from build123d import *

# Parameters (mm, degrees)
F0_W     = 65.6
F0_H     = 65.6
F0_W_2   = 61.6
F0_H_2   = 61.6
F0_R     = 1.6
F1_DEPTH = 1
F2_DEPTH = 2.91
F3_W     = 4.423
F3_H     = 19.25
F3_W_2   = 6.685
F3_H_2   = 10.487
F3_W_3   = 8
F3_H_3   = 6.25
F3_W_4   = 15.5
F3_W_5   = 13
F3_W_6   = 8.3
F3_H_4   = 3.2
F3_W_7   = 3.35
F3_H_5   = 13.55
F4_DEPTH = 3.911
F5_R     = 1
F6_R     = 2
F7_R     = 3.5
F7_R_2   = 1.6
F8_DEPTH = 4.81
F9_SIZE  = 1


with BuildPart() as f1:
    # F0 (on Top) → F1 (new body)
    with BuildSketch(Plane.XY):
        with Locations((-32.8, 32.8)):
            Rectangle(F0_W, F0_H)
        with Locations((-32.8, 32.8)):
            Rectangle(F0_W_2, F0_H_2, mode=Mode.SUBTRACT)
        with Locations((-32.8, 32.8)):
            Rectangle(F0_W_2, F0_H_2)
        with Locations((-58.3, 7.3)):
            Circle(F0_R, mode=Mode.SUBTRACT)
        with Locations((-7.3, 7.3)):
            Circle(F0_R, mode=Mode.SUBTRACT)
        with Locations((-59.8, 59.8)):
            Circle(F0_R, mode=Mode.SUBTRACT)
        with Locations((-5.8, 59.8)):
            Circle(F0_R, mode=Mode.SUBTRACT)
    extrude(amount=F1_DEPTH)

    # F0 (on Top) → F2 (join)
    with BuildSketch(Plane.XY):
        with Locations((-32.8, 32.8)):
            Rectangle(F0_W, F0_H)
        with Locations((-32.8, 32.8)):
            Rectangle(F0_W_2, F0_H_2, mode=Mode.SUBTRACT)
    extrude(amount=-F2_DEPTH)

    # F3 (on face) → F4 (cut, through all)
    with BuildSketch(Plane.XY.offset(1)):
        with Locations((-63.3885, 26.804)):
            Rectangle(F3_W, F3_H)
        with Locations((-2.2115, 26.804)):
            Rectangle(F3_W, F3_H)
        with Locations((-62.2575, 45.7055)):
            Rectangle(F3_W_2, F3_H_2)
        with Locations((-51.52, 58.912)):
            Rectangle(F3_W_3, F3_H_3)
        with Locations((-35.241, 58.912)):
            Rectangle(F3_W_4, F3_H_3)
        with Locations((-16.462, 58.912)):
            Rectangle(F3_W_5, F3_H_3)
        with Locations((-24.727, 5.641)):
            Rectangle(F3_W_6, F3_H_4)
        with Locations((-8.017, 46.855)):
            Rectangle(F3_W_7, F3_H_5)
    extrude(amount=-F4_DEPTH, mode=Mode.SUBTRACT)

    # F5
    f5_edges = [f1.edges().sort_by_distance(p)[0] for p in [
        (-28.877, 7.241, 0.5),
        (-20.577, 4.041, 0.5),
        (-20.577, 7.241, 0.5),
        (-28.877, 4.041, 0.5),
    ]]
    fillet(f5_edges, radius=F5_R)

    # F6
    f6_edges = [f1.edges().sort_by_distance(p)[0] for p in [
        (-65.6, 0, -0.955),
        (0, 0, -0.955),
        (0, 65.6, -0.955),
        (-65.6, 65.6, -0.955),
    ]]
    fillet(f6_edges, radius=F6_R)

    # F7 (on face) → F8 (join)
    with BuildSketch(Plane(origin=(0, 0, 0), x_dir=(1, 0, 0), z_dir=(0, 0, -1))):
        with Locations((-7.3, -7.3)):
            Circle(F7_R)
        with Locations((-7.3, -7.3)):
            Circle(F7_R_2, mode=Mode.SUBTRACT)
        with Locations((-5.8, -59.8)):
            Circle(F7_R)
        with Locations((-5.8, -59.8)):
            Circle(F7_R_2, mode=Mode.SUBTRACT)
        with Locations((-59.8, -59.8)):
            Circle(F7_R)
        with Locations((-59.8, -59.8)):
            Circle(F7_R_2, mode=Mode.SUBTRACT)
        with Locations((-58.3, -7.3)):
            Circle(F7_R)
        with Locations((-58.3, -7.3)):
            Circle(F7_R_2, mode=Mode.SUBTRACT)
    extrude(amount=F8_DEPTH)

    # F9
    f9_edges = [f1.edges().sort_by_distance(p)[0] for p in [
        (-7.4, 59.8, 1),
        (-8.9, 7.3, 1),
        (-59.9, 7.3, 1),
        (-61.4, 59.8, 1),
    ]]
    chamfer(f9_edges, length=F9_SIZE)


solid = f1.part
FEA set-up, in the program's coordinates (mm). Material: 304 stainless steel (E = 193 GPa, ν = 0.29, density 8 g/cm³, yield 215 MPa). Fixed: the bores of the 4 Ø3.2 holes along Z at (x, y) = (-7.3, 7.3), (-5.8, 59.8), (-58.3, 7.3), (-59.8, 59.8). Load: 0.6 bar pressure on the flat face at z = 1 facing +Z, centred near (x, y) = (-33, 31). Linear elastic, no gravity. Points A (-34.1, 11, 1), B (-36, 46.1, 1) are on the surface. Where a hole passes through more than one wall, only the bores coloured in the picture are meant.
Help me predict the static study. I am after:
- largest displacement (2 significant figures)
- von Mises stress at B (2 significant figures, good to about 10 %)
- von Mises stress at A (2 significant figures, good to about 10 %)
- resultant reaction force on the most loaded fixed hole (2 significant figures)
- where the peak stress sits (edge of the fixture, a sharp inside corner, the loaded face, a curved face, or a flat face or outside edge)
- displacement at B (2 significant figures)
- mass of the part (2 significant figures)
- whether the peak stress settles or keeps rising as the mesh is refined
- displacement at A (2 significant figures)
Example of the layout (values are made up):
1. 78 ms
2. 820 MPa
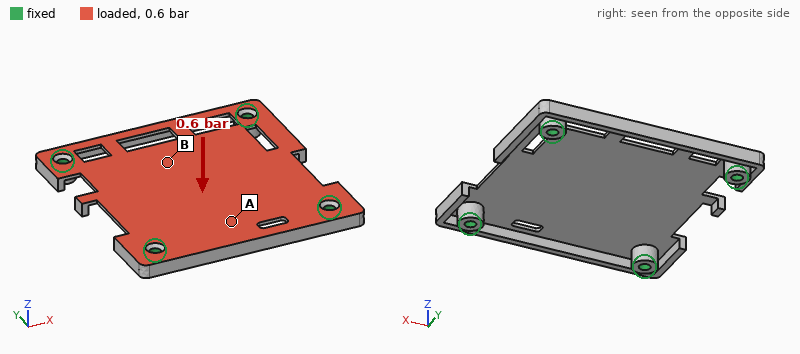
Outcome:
1. 0.13 mm
2. 37 MPa
3. 21 MPa
4. 70 N
5. a sharp inside corner
6. 0.10 mm
7. 44 g
8. keeps rising
9. 0.047 mm
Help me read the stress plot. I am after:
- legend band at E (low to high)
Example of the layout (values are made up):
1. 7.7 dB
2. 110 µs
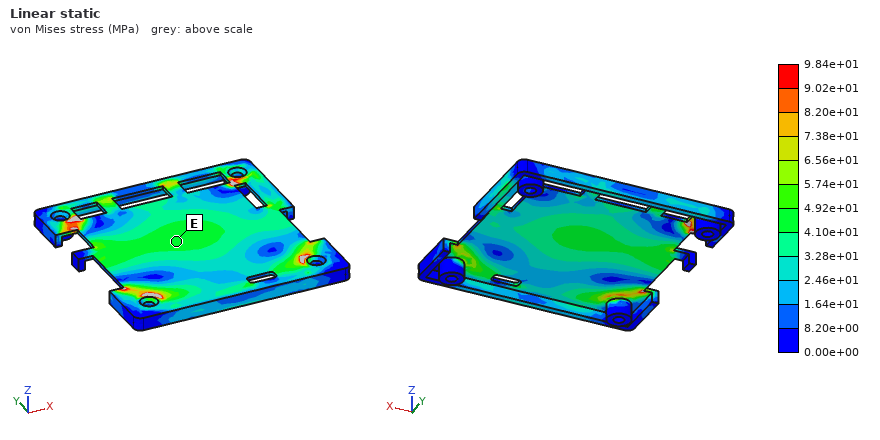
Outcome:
1. 4.10e+01 to 4.92e+01 MPa
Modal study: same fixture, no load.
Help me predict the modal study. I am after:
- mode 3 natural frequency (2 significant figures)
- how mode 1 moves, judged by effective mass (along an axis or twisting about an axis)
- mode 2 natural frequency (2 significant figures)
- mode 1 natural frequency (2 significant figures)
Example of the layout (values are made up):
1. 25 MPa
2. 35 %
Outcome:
1. 3300 Hz
2. along Z
3. 2500 Hz
4. 1500 Hz
